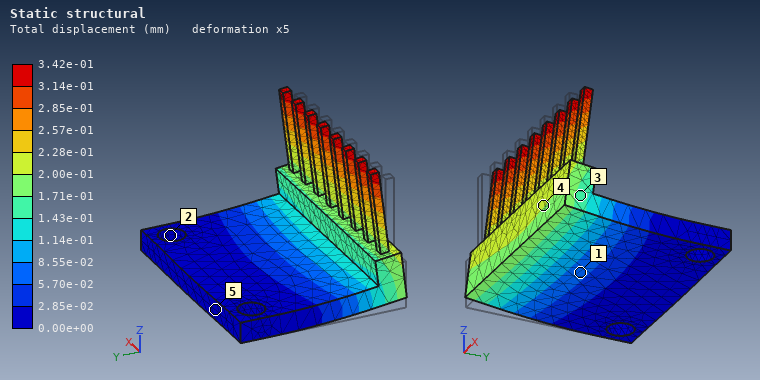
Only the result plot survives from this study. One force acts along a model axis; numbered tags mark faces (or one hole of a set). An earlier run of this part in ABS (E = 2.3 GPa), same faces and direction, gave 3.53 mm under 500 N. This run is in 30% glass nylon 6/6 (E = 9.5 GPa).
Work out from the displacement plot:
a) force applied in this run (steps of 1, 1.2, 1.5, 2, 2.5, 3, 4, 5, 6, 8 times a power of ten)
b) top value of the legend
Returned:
200 N
3.42e-01 mm
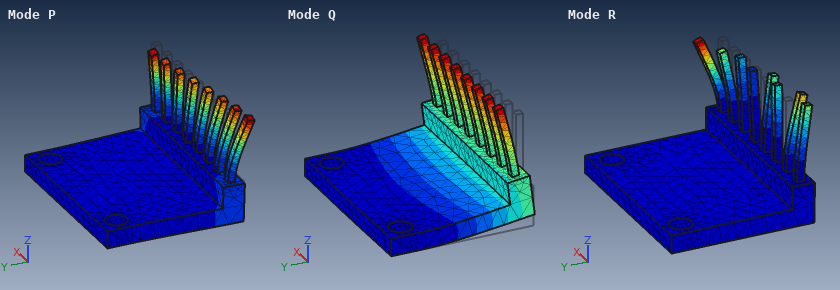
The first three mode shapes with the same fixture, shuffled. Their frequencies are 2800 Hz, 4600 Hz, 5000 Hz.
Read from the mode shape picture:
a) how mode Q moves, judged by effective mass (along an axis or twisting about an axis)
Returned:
along Z
